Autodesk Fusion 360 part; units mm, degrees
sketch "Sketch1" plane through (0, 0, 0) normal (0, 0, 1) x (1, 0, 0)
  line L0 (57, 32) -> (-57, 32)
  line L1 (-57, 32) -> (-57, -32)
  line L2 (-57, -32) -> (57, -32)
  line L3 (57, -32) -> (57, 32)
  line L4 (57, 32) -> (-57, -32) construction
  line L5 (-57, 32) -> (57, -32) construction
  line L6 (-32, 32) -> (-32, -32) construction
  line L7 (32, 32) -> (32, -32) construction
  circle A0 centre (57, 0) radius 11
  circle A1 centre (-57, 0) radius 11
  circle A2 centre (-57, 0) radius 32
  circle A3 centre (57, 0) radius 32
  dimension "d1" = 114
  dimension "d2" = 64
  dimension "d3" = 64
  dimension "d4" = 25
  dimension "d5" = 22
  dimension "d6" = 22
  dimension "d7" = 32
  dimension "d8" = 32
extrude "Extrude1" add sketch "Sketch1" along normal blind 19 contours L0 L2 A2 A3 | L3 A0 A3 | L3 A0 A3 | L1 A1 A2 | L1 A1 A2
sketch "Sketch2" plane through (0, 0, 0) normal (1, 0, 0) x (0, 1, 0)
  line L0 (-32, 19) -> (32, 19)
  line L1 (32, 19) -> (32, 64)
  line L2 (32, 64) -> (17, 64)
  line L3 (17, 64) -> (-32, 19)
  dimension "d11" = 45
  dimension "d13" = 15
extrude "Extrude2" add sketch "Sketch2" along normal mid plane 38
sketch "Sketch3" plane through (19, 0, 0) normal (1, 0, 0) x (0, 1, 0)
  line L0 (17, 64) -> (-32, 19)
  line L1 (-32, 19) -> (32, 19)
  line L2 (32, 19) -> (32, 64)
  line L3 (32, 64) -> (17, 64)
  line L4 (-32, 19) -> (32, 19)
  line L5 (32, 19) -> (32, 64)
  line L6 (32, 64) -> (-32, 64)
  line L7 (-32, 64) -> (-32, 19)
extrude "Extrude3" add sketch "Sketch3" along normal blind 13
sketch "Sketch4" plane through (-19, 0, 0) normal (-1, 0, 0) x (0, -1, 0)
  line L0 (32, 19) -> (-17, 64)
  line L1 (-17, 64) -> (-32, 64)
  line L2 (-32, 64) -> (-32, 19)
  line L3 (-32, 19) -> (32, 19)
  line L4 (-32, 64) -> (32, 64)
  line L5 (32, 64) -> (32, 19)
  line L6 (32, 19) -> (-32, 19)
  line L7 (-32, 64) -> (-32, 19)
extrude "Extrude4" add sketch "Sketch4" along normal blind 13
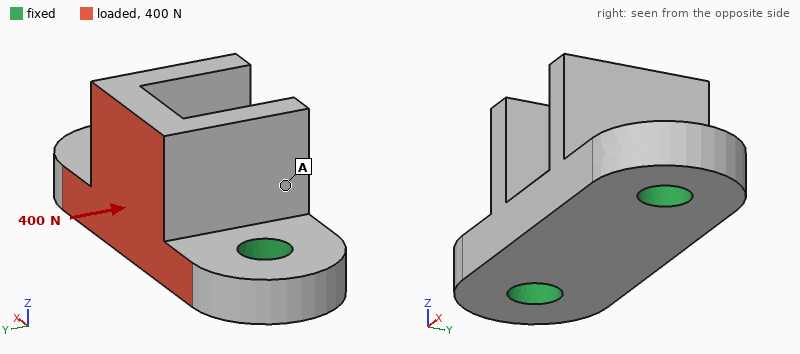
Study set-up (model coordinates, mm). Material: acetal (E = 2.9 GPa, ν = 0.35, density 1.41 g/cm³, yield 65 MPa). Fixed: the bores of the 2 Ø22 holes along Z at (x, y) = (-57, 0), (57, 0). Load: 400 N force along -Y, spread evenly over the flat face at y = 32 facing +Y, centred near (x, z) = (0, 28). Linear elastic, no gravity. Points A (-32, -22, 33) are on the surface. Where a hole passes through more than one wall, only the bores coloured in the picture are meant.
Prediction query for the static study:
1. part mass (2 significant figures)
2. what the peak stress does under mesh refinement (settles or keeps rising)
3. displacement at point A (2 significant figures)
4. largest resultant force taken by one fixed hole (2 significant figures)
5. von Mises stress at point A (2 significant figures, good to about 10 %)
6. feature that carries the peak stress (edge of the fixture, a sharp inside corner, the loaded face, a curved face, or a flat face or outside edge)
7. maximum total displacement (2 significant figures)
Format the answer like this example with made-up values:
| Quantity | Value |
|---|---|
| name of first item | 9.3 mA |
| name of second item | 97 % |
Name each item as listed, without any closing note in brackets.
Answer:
| Quantity | Value |
|---|---|
| part mass | 460 g |
| what the peak stress does under mesh refinement | keeps rising |
| displacement at point A | 21 µm |
| largest resultant force taken by one fixed hole | 200 N |
| von Mises stress at point A | 0.20 MPa |
| feature that carries the peak stress | edge of the fixture |
| maximum total displacement | 42 µm |
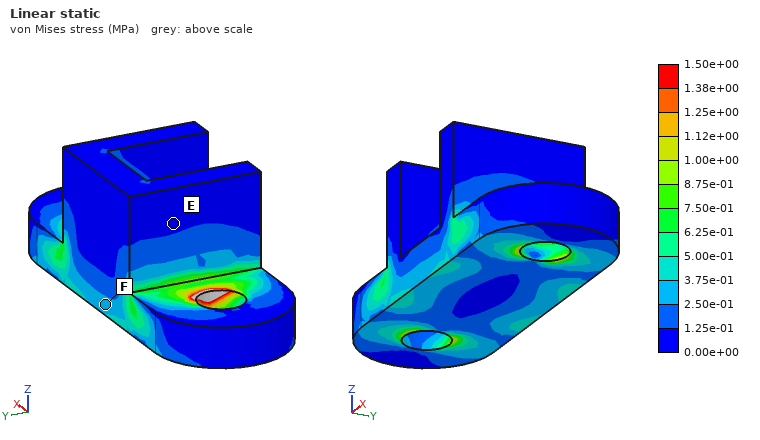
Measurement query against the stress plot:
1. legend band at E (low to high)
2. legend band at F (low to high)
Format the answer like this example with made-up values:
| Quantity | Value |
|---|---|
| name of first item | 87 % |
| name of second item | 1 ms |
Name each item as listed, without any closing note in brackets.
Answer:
| Quantity | Value |
|---|---|
| legend band at E | 0.00e+00 to 1.25e-01 MPa |
| legend band at F | 2.50e-01 to 3.75e-01 MPa |
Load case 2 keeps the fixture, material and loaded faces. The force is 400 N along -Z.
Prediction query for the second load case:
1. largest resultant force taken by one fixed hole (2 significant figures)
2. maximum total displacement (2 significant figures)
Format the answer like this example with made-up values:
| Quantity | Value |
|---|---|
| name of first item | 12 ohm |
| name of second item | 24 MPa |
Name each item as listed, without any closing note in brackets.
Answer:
| Quantity | Value |
|---|---|
| largest resultant force taken by one fixed hole | 210 N |
| maximum total displacement | 61 µm |
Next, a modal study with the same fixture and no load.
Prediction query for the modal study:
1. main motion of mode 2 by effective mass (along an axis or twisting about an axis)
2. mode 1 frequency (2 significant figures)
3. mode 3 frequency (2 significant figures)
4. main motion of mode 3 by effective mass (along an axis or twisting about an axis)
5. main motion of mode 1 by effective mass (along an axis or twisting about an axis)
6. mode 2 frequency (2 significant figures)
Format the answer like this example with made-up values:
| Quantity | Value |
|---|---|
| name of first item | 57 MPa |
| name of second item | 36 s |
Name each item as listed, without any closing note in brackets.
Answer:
| Quantity | Value |
|---|---|
| main motion of mode 2 by effective mass | along Z |
| mode 1 frequency | 980 Hz |
| mode 3 frequency | 2000 Hz |
| main motion of mode 3 by effective mass | along X |
| main motion of mode 1 by effective mass | along Y |
| mode 2 frequency | 1800 Hz |
